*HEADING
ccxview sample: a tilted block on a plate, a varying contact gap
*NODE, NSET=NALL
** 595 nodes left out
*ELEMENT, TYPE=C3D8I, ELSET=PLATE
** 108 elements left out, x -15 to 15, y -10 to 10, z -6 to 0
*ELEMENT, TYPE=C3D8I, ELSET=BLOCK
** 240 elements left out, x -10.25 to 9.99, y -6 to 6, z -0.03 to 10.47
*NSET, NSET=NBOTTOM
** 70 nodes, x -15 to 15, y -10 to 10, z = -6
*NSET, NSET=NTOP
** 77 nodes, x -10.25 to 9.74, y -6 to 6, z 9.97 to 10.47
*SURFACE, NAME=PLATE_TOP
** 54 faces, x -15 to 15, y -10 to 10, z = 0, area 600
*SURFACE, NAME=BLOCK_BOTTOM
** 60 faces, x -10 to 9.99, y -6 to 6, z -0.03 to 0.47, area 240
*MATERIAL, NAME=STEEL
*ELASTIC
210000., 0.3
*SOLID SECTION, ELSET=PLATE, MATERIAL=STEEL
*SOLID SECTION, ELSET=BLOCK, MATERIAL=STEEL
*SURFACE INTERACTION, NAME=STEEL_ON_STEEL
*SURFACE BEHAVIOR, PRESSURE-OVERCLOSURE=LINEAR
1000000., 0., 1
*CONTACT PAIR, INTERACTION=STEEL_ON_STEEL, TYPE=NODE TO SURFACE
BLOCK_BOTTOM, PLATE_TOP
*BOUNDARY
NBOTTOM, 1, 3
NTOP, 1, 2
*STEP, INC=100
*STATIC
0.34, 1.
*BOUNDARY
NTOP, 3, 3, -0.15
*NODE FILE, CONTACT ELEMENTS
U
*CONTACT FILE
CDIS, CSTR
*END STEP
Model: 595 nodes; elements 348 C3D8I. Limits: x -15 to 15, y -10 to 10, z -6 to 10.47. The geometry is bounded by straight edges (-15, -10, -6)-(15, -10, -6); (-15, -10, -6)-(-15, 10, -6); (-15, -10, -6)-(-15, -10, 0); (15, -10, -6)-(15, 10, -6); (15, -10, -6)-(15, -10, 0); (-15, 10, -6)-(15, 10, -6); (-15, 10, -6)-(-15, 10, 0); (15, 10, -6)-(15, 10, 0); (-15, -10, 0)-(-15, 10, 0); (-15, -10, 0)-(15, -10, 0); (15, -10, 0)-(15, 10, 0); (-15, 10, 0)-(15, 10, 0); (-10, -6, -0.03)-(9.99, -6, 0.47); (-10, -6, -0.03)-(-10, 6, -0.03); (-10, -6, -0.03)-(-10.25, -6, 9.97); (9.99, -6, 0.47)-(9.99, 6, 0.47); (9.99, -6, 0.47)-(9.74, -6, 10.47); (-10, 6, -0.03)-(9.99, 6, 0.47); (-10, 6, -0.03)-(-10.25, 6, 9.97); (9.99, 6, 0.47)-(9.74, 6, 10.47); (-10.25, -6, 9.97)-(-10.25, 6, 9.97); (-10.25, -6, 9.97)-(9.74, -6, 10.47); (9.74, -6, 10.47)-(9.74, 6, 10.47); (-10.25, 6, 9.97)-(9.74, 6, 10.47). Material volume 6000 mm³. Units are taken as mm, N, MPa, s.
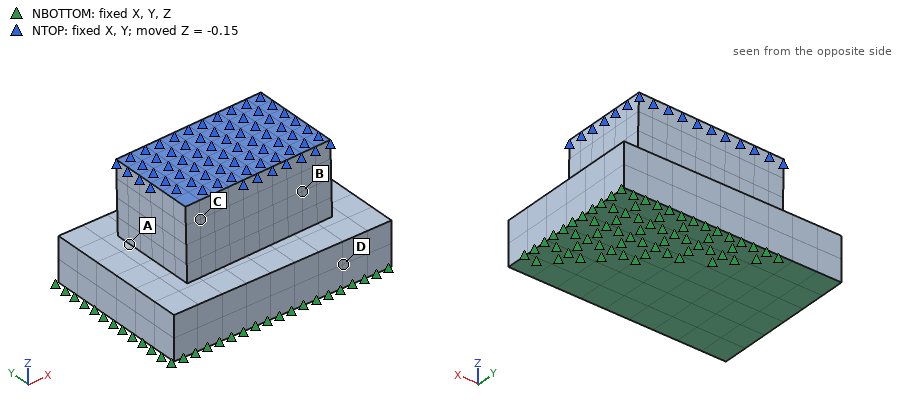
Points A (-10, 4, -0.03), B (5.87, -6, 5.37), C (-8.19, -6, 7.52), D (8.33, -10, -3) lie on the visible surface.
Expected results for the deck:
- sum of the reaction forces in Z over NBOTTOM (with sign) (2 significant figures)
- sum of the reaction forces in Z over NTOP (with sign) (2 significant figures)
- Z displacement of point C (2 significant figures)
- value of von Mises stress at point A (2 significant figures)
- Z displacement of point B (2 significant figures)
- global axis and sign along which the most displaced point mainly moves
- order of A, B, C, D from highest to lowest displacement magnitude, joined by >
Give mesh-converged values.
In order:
1.3e+05 N
-1.3e+05 N
-0.13 mm
4900 MPa
-0.15 mm
-Z
B > C > A > D
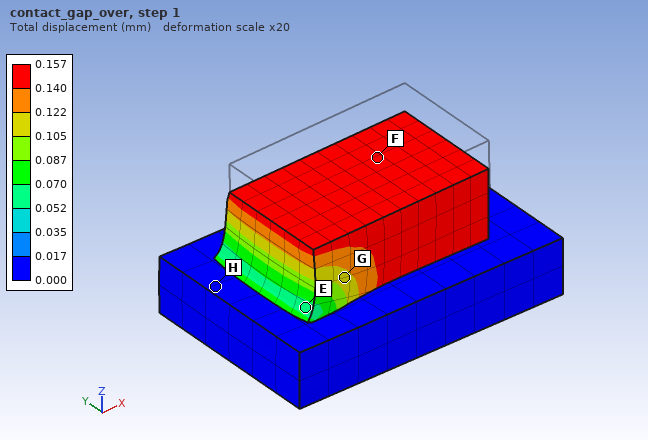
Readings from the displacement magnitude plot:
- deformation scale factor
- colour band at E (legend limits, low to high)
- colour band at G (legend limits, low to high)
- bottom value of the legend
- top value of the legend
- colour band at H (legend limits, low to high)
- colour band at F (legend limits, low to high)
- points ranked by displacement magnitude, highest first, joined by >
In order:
20
0.052 to 0.070 mm
0.105 to 0.122 mm
0.000 mm
0.157 mm
0.000 to 0.017 mm
0.140 to 0.157 mm
F > G > E > H
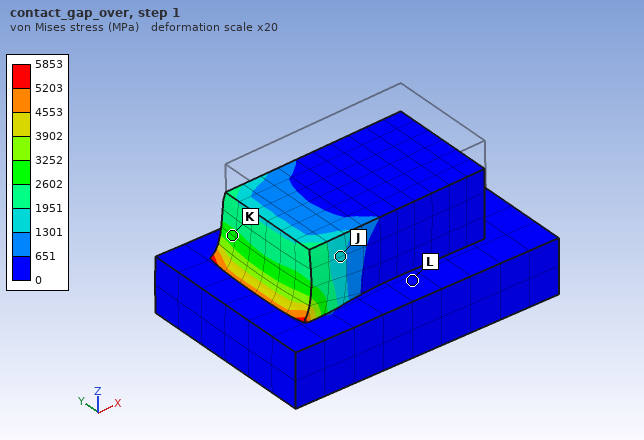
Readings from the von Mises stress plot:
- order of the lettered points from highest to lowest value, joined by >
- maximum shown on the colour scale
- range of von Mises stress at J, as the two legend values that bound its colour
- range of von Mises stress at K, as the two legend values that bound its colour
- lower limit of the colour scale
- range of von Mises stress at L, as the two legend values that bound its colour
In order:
K > J > L
5853 MPa
1301 to 1951 MPa
2602 to 3252 MPa
0 MPa
0 to 651 MPa
